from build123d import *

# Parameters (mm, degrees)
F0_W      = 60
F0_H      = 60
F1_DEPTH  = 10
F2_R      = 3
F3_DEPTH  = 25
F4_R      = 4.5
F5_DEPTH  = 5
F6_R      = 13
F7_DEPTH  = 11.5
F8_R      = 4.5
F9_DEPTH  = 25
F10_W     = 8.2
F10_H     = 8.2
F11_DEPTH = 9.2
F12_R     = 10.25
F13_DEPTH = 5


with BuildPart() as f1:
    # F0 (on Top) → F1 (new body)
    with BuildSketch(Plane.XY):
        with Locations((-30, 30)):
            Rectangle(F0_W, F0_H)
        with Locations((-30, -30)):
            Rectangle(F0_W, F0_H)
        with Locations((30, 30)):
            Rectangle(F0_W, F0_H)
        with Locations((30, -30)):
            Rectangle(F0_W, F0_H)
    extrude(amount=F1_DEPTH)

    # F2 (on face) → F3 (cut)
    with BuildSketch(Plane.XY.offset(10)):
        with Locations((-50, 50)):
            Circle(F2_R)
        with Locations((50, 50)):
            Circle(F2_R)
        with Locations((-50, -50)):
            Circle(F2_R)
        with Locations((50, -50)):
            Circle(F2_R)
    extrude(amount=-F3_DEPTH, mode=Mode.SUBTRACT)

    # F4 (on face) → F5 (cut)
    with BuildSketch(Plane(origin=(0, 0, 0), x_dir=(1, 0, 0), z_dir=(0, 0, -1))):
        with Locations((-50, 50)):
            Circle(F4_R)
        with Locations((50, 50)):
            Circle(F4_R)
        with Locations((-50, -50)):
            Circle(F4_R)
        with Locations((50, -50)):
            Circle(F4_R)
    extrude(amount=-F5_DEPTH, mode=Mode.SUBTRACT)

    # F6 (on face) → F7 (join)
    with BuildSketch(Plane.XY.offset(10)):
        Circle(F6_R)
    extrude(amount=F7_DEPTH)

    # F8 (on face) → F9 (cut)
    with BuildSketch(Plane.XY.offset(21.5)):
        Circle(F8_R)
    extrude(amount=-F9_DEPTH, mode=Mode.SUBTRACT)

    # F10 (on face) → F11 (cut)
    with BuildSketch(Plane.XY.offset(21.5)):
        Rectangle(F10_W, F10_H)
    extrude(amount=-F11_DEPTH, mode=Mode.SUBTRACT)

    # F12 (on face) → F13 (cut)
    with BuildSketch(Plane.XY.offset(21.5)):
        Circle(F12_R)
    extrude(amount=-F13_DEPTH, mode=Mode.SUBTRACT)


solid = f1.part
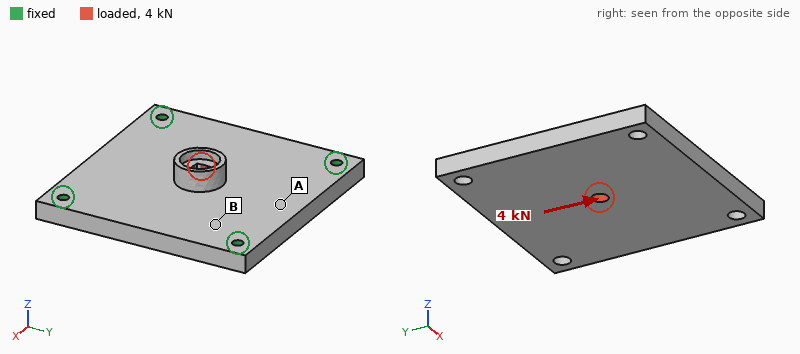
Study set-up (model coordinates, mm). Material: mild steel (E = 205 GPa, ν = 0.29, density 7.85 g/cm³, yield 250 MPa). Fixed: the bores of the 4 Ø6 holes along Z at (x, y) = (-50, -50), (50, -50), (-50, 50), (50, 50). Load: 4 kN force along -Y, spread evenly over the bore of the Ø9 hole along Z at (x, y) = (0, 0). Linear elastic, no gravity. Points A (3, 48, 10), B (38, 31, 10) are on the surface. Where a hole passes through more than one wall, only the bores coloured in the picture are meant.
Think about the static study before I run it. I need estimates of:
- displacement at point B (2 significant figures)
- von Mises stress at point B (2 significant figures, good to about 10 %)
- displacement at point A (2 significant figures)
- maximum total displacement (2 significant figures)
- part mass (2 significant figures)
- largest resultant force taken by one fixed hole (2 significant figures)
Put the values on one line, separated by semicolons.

1.1 µm; 5.4 MPa; 2.0 µm; 3.4 µm; 1.1 kg; 1.1 kN
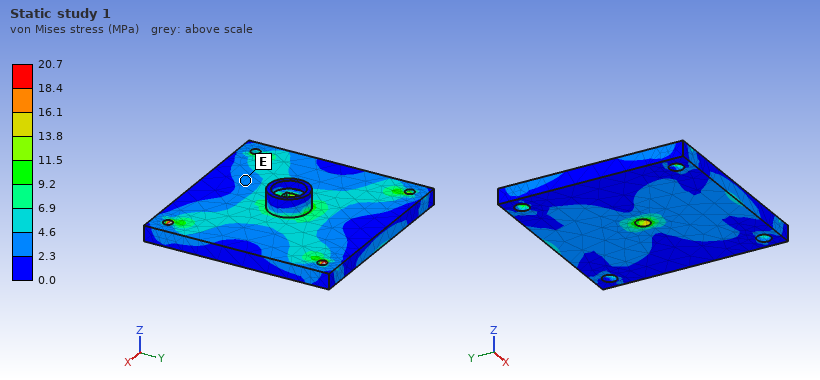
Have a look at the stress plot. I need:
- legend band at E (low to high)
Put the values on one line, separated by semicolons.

2.3 to 4.6 MPa
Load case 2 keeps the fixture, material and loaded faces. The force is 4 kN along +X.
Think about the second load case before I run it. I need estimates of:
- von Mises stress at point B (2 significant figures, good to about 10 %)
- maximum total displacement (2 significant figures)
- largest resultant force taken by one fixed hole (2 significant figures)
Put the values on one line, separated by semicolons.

4.9 MPa; 3.4 µm; 1.1 kN
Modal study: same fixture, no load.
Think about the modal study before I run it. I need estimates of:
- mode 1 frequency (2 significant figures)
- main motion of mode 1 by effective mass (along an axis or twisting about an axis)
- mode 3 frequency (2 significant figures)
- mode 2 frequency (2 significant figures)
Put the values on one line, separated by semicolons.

2600 Hz; along Z; 4500 Hz; 4500 Hz
